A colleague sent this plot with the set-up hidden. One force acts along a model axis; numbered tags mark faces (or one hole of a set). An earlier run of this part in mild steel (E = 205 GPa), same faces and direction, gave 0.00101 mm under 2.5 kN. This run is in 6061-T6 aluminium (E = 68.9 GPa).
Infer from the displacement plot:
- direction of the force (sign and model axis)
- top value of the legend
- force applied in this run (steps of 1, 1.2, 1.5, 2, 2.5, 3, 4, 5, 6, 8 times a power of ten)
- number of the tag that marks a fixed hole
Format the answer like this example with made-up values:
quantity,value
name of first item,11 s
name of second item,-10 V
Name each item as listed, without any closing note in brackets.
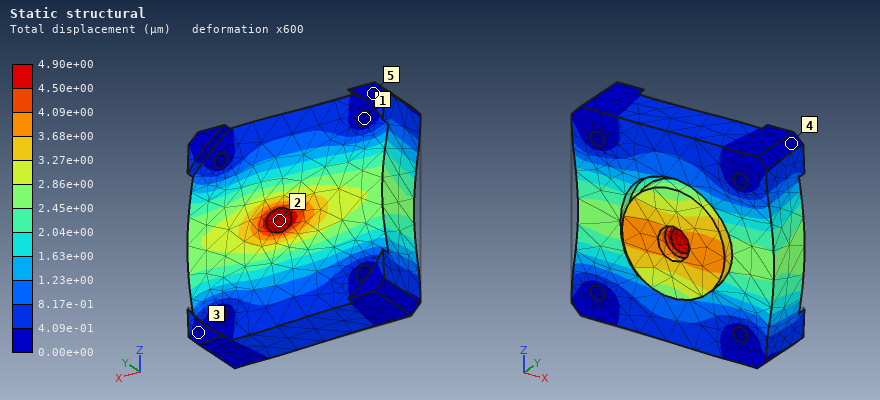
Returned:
quantity,value
direction of the force,+X
top value of the legend,4.90e+00 µm
force applied in this run,4 kN
number of the tag that marks a fixed hole,1
